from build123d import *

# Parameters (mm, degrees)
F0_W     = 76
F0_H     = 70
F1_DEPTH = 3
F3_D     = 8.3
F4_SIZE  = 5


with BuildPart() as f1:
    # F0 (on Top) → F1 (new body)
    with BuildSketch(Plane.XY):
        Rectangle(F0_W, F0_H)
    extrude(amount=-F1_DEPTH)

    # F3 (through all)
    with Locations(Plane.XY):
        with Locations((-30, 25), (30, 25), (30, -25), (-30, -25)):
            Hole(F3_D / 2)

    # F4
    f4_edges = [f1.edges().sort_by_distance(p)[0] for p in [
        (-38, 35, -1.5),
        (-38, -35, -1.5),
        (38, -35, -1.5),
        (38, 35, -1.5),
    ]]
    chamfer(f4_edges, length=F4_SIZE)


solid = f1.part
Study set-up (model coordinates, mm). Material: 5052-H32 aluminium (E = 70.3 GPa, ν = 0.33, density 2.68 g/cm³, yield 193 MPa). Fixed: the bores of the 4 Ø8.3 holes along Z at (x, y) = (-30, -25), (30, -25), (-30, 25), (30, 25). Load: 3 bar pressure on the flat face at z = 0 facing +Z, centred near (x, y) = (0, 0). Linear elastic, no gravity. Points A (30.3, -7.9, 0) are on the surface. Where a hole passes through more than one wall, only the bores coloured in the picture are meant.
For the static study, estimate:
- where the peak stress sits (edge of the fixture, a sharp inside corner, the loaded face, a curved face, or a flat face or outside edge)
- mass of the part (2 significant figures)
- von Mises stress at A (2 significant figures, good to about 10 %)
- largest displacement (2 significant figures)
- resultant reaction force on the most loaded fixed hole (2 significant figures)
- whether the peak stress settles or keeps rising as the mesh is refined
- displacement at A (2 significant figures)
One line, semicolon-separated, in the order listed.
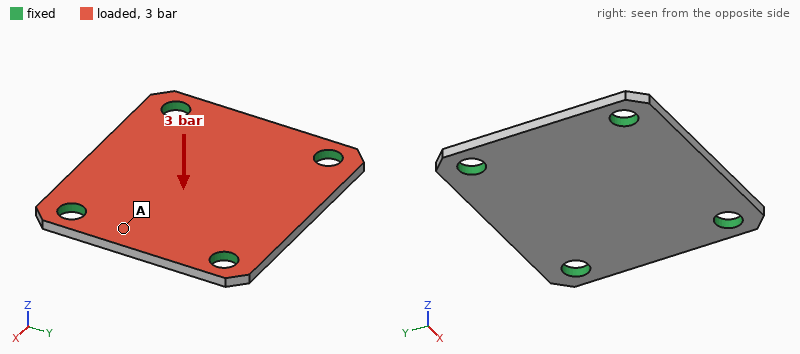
edge of the fixture; 41 g; 16 MPa; 78 µm; 380 N; keeps rising; 19 µm
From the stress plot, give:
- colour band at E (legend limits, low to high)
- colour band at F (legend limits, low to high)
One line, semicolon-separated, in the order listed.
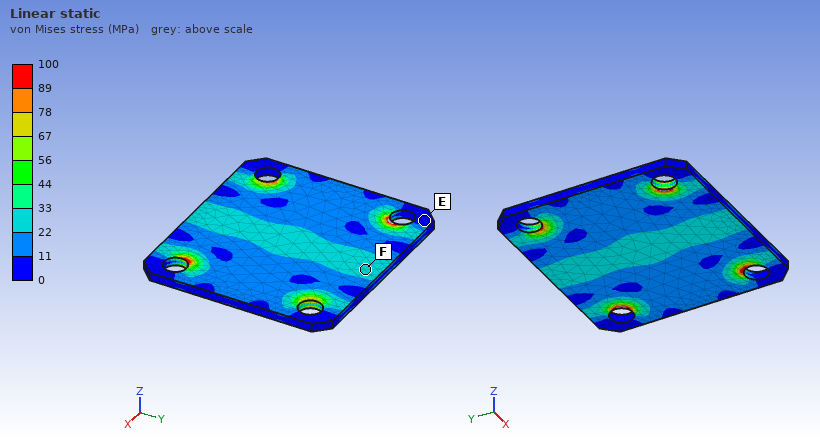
0 to 11 MPa; 22 to 33 MPa
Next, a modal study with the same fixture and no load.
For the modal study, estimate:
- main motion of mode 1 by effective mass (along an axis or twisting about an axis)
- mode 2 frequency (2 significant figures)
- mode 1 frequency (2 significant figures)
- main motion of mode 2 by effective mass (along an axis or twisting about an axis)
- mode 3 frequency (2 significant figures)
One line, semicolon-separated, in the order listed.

along Z; 5900 Hz; 4300 Hz; twisting about X; 6900 Hz
